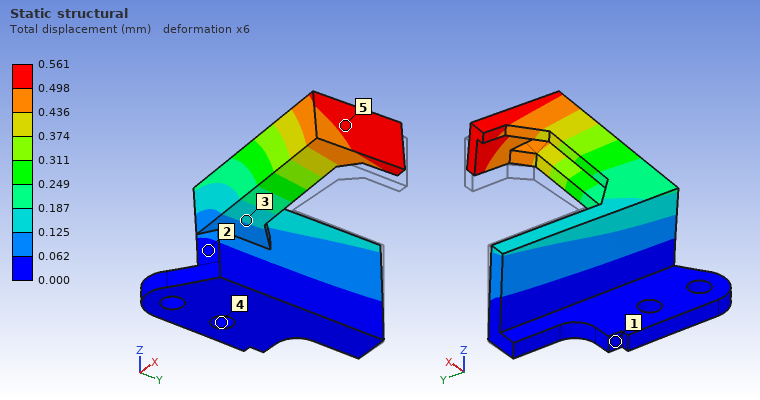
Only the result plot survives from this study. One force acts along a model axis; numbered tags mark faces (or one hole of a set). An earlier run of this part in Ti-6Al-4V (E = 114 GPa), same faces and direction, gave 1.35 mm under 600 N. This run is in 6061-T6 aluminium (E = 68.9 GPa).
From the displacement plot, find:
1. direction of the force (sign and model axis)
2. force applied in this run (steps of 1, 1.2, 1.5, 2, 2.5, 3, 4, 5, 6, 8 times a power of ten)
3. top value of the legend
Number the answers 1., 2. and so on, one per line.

1. +Z
2. 150 N
3. 0.561 mm
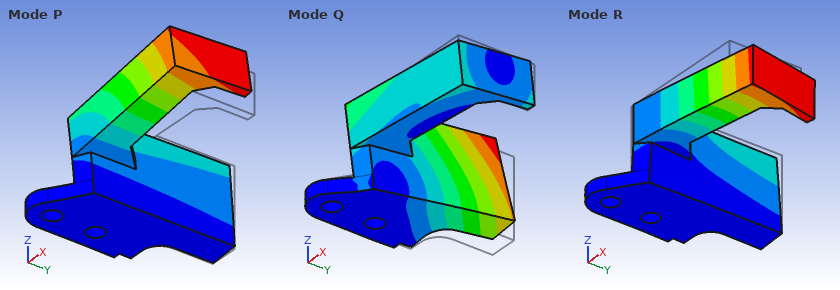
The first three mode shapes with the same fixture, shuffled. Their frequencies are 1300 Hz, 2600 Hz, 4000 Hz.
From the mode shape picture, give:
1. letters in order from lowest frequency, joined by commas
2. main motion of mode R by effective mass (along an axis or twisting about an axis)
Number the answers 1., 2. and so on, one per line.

1. P, R, Q
2. along Y
